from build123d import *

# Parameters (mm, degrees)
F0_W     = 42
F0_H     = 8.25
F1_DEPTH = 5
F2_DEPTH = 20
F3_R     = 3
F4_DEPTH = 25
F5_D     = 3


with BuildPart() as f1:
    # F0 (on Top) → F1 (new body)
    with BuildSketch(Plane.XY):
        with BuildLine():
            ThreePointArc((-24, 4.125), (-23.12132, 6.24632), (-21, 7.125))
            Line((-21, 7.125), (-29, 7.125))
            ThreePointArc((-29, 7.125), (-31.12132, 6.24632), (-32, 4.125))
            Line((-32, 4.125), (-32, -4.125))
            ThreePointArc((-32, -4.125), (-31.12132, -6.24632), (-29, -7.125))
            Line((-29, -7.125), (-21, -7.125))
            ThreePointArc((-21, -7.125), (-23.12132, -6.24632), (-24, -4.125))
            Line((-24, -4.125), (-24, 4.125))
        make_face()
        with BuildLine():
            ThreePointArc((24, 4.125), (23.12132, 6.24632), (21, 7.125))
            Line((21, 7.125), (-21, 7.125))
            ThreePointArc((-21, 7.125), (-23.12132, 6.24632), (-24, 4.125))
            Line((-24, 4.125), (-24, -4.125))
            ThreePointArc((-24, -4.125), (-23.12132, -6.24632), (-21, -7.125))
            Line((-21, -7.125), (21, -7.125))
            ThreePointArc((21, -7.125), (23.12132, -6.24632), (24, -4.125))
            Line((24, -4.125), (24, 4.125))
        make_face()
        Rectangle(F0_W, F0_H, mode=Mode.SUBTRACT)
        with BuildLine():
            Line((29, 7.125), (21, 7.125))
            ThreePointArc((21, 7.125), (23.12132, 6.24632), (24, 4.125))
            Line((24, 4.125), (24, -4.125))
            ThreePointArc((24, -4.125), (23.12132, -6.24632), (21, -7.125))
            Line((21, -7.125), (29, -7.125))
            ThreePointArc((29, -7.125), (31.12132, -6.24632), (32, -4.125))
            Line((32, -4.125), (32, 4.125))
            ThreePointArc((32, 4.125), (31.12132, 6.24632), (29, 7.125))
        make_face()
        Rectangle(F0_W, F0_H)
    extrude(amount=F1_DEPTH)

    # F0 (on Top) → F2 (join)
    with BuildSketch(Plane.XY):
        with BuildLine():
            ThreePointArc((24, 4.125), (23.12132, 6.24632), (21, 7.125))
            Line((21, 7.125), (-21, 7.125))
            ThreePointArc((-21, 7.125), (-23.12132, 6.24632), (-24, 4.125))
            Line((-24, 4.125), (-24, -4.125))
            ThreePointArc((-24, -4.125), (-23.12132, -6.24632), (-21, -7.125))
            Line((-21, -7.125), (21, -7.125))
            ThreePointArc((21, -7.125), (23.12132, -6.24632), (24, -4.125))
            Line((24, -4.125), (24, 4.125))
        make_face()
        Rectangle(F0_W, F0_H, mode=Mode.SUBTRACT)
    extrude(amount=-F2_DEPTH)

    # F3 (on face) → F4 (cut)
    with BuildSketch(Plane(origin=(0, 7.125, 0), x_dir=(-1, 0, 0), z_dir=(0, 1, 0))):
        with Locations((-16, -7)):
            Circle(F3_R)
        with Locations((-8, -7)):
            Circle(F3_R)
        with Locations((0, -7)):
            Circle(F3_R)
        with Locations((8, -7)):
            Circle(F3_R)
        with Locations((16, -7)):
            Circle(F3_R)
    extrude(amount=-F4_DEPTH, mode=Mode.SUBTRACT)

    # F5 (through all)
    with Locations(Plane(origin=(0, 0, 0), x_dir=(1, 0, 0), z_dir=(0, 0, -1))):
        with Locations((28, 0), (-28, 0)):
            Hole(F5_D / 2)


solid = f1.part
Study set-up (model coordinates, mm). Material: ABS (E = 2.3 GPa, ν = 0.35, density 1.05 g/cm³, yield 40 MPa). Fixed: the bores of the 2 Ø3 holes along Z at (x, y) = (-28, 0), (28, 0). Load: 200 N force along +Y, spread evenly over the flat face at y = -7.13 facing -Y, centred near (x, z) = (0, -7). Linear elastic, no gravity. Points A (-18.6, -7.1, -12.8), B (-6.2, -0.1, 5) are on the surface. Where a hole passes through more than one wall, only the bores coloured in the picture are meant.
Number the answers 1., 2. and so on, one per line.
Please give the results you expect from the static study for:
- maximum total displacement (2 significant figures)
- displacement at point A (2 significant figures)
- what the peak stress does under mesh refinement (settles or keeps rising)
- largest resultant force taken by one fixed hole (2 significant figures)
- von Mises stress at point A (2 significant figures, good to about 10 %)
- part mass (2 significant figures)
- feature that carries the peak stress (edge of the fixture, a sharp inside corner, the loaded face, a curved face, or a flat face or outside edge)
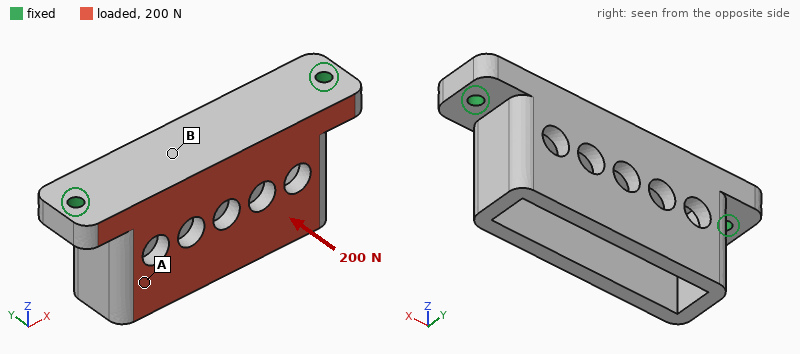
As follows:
1. 0.80 mm
2. 0.33 mm
3. keeps rising
4. 100 N
5. 6.4 MPa
6. 11 g
7. edge of the fixture
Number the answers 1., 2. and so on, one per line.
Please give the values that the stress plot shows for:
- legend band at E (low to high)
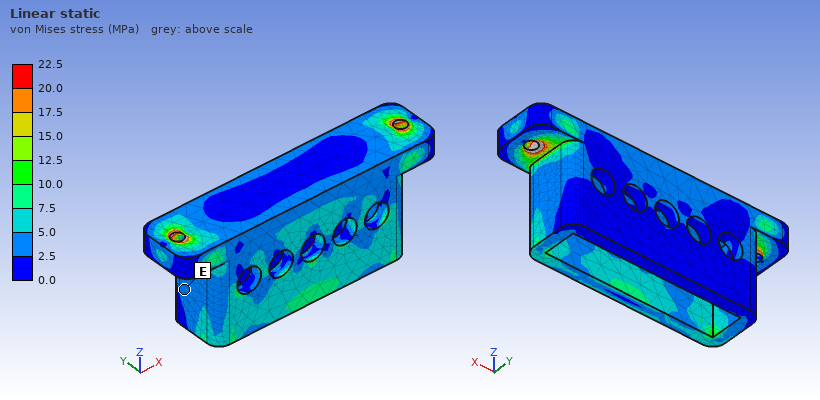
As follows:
1. 2.5 to 5.0 MPa
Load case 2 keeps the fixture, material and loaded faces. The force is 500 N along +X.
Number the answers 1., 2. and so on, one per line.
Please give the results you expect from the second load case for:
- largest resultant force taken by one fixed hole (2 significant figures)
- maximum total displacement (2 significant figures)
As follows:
1. 270 N
2. 0.14 mm
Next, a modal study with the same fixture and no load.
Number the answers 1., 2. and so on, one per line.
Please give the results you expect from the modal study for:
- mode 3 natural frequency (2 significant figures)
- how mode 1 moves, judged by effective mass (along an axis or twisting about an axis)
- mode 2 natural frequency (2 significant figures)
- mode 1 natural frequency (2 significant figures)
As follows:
1. 2600 Hz
2. along Y
3. 2500 Hz
4. 1300 Hz
